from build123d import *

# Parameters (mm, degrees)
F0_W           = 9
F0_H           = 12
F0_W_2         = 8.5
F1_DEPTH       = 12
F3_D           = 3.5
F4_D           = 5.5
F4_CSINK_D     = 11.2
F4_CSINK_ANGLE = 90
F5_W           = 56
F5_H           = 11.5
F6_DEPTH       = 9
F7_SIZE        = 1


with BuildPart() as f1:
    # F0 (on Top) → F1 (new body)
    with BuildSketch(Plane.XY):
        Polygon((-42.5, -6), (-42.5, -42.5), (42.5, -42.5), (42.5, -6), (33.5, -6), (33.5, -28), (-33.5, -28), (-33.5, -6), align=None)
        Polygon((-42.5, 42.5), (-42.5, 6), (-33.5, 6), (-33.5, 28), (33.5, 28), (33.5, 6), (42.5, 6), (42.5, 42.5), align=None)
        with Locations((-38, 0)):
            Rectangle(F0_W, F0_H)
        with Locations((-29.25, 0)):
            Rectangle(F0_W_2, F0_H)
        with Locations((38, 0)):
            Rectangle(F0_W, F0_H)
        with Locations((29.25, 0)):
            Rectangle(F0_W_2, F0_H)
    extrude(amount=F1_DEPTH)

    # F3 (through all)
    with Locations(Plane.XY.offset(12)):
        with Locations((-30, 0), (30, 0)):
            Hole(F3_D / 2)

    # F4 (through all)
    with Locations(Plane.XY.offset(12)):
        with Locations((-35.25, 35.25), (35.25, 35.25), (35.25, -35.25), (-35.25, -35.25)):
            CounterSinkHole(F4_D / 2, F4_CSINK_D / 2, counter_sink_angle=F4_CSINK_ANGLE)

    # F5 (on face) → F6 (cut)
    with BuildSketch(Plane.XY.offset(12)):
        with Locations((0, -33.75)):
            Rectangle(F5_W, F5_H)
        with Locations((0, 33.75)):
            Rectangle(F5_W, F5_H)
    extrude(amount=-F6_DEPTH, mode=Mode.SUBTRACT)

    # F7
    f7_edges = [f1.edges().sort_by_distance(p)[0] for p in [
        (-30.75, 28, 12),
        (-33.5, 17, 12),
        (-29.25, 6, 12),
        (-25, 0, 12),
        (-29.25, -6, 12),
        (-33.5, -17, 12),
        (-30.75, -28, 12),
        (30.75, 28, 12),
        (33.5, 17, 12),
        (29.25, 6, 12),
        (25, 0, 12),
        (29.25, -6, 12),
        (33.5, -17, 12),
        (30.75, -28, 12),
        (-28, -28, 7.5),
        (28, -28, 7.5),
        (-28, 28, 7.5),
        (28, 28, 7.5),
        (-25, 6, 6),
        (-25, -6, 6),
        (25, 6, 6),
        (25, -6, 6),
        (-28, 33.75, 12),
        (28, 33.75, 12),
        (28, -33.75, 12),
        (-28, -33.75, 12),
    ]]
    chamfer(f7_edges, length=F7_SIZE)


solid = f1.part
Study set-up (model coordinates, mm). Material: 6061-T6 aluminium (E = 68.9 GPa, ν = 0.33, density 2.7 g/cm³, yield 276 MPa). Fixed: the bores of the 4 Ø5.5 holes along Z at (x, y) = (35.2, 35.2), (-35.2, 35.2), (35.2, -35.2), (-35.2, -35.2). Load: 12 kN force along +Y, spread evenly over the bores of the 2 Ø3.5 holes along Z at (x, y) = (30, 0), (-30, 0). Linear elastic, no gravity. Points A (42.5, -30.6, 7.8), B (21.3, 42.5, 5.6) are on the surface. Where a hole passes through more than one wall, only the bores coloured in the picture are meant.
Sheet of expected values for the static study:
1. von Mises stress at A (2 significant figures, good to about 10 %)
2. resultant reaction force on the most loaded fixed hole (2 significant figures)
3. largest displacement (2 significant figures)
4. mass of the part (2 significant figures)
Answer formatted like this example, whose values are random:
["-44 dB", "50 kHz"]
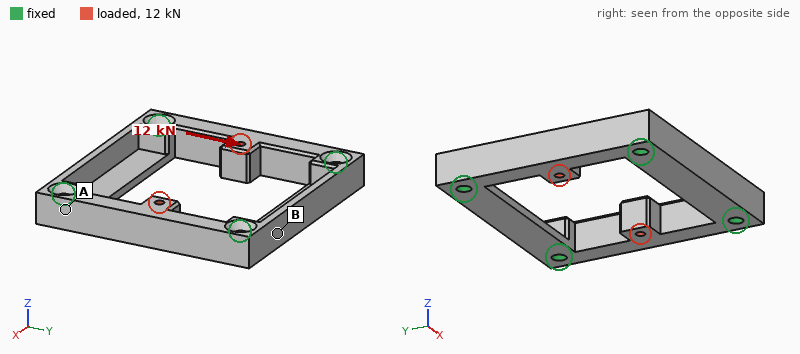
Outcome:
["45 MPa", "3.2 kN", "75 µm", "83 g"]
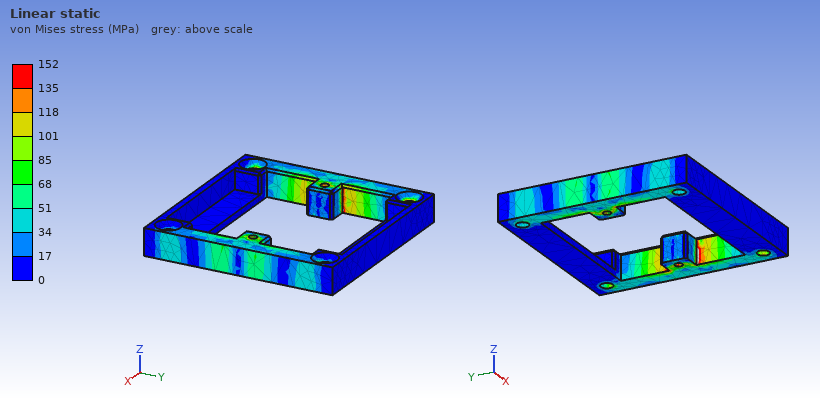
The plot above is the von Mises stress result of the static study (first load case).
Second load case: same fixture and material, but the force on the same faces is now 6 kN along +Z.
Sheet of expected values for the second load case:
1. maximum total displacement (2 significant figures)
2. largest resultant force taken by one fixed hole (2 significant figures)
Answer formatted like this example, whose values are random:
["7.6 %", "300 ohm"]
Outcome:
["0.20 mm", "1.5 kN"]
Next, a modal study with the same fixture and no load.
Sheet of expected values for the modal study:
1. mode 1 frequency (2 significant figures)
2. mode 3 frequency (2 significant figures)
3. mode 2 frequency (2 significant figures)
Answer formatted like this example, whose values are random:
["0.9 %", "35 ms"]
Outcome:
["7600 Hz", "8200 Hz", "7600 Hz"]
